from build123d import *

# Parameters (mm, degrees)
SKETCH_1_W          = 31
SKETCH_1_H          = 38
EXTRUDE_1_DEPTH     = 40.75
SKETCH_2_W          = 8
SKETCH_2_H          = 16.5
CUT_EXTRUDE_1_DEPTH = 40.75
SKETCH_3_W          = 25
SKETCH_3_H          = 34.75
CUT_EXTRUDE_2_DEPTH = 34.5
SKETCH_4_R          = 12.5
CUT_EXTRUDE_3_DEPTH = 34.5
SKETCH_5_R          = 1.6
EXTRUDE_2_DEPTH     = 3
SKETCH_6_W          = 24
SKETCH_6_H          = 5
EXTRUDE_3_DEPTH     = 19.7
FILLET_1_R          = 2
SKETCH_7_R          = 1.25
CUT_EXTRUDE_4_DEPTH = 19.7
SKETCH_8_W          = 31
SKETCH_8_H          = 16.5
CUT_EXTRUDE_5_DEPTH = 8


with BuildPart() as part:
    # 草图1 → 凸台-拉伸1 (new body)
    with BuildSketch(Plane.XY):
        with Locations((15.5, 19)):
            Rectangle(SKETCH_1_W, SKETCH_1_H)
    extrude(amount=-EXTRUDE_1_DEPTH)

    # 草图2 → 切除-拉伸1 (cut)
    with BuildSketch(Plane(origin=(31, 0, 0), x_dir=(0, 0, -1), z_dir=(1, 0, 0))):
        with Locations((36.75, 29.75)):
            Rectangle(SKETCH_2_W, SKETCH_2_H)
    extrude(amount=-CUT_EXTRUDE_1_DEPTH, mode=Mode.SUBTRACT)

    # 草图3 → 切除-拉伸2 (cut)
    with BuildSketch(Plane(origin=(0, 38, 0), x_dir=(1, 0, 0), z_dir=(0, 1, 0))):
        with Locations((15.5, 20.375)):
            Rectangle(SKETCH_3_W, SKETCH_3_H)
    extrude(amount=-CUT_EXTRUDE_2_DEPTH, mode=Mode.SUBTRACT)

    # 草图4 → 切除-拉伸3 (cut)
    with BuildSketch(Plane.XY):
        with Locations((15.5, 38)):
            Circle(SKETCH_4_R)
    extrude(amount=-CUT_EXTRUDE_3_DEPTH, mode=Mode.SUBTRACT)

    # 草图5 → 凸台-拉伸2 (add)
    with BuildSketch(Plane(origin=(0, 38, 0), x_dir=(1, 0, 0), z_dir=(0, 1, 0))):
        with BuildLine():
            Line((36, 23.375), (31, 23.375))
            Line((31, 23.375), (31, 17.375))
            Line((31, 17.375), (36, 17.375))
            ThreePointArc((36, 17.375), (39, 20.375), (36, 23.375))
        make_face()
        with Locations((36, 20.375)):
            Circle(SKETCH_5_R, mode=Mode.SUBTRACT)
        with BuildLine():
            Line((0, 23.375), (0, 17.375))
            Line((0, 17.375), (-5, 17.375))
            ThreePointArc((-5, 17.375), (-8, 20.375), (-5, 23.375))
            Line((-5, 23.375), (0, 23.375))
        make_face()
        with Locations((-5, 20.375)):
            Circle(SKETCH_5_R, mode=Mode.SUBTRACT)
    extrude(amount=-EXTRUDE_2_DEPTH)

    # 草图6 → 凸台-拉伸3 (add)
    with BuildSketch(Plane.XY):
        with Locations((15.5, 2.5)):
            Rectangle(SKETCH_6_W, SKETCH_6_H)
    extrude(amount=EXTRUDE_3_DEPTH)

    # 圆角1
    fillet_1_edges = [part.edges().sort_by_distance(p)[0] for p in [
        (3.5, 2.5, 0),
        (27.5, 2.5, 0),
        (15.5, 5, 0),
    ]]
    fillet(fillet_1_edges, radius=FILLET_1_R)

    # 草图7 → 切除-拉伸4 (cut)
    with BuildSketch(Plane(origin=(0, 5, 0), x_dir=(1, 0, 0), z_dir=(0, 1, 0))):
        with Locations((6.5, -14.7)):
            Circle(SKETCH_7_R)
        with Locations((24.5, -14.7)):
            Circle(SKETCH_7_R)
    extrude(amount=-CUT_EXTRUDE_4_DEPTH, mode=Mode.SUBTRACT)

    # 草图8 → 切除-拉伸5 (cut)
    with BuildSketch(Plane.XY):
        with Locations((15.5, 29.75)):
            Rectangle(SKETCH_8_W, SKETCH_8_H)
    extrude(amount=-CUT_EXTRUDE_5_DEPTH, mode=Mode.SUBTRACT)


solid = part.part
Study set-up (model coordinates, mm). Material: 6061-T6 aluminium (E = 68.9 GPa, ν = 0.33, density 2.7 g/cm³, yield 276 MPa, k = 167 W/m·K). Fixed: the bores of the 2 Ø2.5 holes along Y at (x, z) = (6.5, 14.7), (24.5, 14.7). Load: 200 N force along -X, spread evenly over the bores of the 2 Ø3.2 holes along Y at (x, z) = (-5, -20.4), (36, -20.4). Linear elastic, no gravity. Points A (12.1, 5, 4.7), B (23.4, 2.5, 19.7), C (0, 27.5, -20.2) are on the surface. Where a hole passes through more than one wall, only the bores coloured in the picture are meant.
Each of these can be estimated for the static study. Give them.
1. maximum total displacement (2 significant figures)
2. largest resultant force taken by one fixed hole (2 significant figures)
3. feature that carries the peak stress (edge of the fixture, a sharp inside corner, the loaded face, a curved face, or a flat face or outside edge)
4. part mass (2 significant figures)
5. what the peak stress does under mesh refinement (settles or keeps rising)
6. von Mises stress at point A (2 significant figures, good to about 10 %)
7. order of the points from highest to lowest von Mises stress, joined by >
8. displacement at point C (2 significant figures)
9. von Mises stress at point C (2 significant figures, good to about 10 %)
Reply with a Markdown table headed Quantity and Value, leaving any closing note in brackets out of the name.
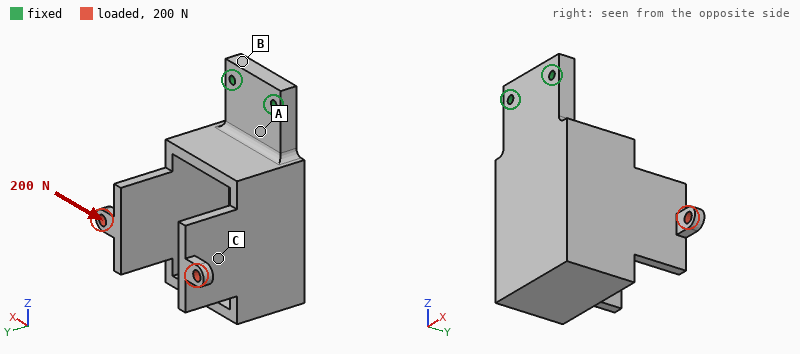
| Quantity | Value |
|---|---|
| maximum total displacement | 0.34 mm |
| largest resultant force taken by one fixed hole | 530 N |
| feature that carries the peak stress | edge of the fixture |
| part mass | 45 g |
| what the peak stress does under mesh refinement | keeps rising |
| von Mises stress at point A | 45 MPa |
| order of the points from highest to lowest von Mises stress, joined by > | A > C > B |
| displacement at point C | 0.19 mm |
| von Mises stress at point C | 31 MPa |
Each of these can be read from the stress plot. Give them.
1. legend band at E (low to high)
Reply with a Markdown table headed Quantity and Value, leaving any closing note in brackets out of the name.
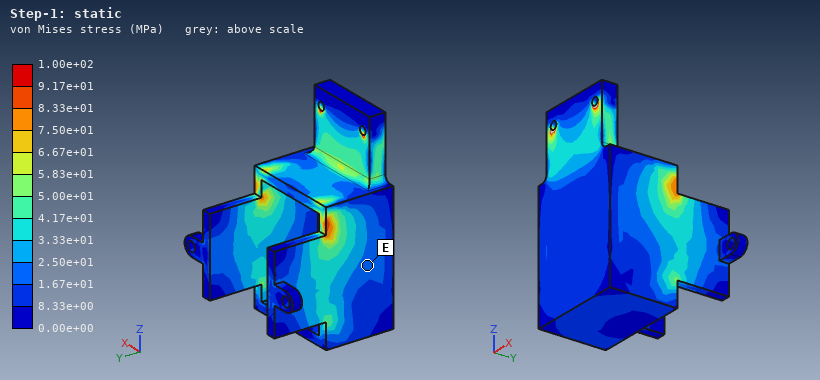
| Quantity | Value |
|---|---|
| legend band at E | 1.67e+01 to 2.50e+01 MPa |
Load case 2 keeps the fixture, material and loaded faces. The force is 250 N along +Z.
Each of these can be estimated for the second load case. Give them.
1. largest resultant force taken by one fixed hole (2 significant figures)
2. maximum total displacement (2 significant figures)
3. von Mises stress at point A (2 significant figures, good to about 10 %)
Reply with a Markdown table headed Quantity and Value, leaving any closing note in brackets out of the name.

| Quantity | Value |
|---|---|
| largest resultant force taken by one fixed hole | 130 N |
| maximum total displacement | 0.51 mm |
| von Mises stress at point A | 73 MPa |
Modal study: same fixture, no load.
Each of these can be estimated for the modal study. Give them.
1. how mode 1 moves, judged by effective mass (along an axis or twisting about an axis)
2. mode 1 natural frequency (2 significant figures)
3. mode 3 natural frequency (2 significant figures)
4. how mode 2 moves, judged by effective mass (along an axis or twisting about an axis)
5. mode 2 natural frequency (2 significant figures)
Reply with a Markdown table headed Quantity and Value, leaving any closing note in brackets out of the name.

| Quantity | Value |
|---|---|
| how mode 1 moves, judged by effective mass | along Y |
| mode 1 natural frequency | 730 Hz |
| mode 3 natural frequency | 3300 Hz |
| how mode 2 moves, judged by effective mass | along X |
| mode 2 natural frequency | 1500 Hz |
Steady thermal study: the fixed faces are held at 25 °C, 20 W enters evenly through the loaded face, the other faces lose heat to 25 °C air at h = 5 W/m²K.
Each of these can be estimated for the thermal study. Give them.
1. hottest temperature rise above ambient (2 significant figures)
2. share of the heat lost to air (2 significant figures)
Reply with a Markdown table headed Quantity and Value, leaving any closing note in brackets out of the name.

| Quantity | Value |
|---|---|
| hottest temperature rise above ambient | 74 K |
| share of the heat lost to air | 7.0 % |
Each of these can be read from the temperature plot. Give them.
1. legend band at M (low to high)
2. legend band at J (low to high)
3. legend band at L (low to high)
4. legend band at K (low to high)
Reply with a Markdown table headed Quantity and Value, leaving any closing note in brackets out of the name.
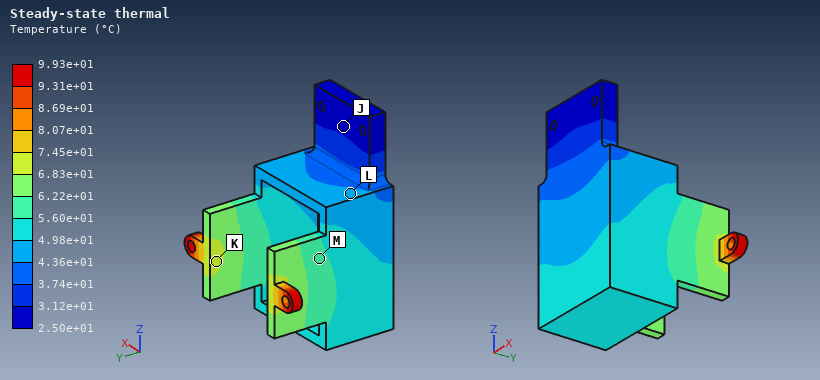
| Quantity | Value |
|---|---|
| legend band at M | 5.60e+01 to 6.22e+01 °C |
| legend band at J | 2.50e+01 to 3.12e+01 °C |
| legend band at L | 4.36e+01 to 4.98e+01 °C |
| legend band at K | 6.83e+01 to 7.45e+01 °C |
